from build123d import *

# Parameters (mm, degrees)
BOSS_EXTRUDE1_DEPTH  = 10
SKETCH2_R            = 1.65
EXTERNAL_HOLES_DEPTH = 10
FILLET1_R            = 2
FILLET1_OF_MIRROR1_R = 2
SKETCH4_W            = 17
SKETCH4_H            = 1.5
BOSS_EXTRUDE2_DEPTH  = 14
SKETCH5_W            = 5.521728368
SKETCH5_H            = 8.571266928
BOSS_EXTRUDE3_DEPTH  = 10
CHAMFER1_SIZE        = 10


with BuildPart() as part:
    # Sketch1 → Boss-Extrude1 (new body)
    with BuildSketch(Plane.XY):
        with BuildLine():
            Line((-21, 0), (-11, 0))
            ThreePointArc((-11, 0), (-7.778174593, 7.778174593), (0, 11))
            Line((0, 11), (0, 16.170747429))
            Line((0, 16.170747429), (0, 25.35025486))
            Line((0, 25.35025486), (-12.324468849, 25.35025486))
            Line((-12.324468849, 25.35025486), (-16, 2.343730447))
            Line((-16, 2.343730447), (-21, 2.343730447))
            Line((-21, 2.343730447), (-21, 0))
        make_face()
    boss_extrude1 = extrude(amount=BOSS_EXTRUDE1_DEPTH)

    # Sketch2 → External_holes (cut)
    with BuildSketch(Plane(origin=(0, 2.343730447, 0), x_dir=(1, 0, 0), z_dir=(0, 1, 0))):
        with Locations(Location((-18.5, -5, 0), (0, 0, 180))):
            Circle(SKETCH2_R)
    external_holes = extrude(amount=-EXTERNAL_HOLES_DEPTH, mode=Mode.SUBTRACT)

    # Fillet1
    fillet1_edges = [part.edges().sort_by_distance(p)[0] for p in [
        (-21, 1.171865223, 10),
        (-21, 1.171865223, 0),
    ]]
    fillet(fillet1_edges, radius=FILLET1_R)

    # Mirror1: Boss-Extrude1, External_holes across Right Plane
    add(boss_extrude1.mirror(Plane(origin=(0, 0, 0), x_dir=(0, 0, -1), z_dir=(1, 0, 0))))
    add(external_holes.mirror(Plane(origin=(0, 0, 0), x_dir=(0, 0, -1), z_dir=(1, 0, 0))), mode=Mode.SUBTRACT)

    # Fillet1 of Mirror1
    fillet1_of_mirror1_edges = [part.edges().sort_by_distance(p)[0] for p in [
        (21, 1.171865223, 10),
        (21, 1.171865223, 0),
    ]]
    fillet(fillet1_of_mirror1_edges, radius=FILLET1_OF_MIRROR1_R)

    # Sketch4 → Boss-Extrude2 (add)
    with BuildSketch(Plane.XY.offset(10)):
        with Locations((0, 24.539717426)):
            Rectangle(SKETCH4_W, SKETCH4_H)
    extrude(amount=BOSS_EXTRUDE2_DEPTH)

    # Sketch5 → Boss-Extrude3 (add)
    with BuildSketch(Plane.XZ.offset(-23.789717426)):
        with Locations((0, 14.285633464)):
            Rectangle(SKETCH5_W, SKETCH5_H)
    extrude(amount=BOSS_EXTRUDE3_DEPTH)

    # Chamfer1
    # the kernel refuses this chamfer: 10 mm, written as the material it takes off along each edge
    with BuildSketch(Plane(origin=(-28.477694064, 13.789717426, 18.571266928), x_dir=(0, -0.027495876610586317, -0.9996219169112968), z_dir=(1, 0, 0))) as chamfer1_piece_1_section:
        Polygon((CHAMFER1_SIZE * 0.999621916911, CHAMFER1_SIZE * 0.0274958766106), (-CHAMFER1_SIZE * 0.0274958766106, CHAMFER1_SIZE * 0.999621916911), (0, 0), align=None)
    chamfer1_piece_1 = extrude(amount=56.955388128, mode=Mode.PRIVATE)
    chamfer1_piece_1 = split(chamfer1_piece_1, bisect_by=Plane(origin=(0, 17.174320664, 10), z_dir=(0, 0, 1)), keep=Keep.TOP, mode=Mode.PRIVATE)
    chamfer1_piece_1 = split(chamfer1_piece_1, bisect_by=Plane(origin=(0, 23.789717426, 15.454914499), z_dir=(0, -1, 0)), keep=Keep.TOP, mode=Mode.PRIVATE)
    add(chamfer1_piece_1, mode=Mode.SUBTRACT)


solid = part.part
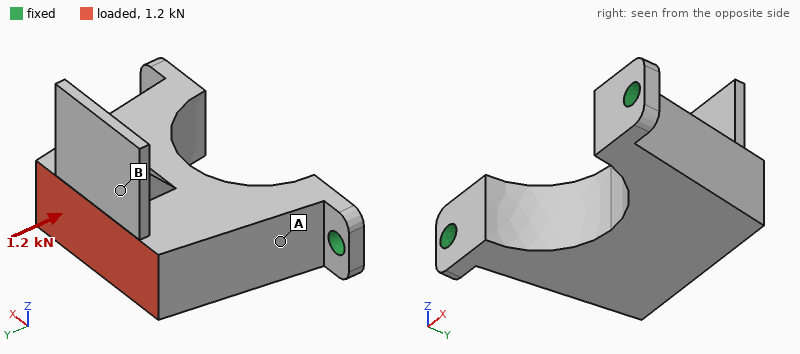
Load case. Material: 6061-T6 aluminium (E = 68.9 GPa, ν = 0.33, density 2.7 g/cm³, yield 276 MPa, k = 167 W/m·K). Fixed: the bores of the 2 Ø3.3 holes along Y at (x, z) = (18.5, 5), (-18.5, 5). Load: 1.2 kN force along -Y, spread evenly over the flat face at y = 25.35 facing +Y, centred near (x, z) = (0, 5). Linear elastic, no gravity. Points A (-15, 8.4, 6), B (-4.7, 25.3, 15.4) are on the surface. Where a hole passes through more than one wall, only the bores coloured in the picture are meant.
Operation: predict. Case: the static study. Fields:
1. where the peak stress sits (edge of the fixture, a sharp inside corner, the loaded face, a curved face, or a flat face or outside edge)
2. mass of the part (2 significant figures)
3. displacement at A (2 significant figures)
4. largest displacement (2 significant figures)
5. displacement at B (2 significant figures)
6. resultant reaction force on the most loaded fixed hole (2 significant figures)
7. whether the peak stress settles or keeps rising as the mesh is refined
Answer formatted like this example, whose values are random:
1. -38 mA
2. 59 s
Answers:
1. edge of the fixture
2. 17 g
3. 7.1 µm
4. 9.1 µm
5. 8.8 µm
6. 700 N
7. keeps rising
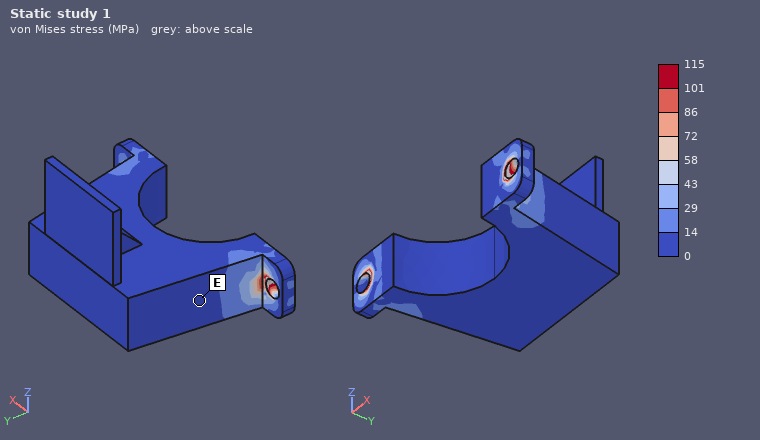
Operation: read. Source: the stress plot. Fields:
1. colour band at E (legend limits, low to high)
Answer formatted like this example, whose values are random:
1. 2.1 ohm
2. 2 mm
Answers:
1. 0 to 14 MPa
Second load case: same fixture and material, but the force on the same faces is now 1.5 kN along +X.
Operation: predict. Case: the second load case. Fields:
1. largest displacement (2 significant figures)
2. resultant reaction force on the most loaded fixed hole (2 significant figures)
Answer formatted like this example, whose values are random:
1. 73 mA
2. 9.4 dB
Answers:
1. 29 µm
2. 1.3 kN
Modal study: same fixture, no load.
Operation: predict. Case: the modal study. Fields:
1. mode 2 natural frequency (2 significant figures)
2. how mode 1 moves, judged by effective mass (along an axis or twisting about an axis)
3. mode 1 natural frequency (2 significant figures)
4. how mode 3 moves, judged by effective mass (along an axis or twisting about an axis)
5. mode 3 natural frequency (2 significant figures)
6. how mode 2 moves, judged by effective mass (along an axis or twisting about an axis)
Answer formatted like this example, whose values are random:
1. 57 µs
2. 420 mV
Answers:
1. 12 kHz
2. along Z
3. 2400 Hz
4. along X
5. 14 kHz
6. along X
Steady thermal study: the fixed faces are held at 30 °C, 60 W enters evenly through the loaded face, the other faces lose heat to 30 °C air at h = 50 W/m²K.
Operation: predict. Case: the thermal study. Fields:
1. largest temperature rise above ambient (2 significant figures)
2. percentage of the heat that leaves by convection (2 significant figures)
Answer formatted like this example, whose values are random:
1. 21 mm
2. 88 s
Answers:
1. 71 K
2. 11 %
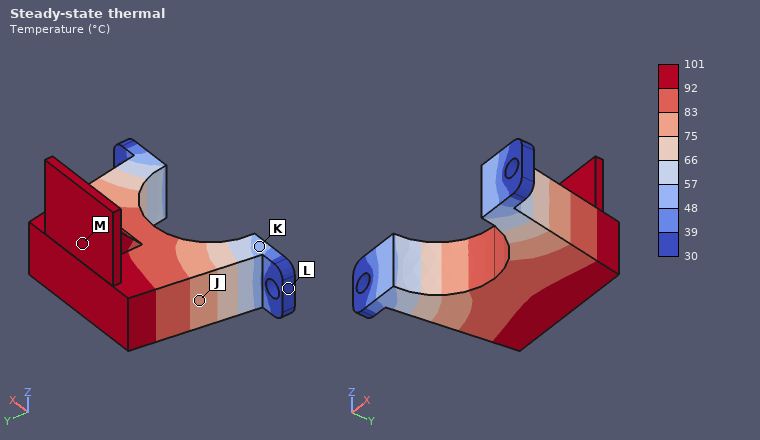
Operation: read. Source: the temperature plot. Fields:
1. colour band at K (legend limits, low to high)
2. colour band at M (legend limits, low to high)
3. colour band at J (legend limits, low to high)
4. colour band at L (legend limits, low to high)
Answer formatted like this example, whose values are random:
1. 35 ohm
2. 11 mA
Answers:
1. 48 to 57 °C
2. 92 to 101 °C
3. 75 to 83 °C
4. 30 to 39 °C
